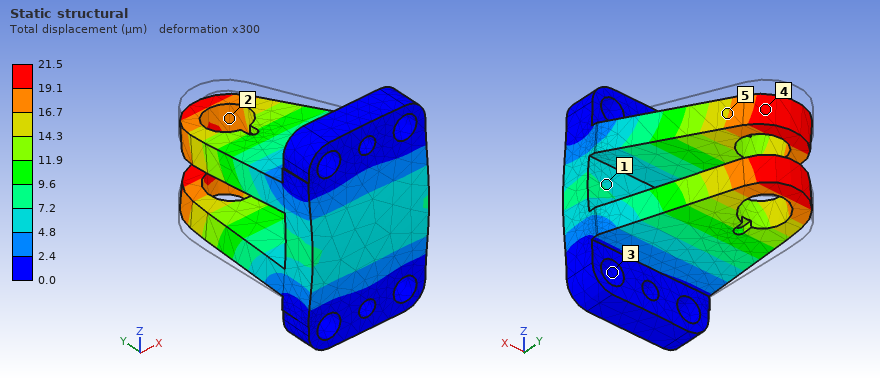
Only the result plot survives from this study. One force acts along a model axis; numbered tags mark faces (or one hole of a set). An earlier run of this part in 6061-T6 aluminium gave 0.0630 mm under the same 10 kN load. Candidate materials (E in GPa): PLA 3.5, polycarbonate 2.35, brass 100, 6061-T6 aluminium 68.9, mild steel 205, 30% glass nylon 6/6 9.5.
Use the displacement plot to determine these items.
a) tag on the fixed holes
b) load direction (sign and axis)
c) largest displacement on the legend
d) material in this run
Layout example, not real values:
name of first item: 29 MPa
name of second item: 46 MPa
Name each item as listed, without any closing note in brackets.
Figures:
tag on the fixed holes: 3
load direction: -Y
largest displacement on the legend: 21.5 µm
material in this run: mild steel
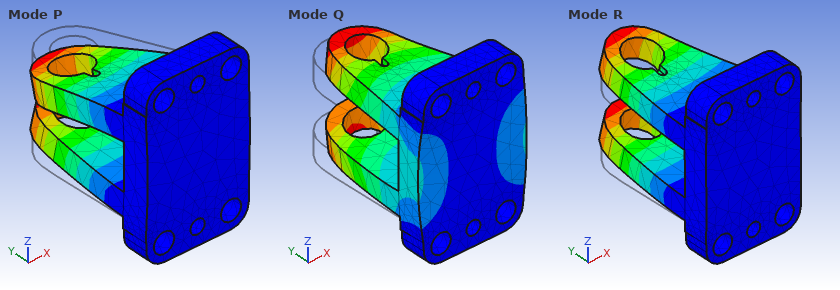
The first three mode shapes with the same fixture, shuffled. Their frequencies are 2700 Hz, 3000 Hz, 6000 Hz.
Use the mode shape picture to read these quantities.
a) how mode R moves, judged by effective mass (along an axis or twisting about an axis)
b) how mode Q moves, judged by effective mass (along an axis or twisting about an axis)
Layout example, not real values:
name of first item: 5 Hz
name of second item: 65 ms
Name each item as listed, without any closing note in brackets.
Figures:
how mode R moves, judged by effective mass: along Z
how mode Q moves, judged by effective mass: along X
